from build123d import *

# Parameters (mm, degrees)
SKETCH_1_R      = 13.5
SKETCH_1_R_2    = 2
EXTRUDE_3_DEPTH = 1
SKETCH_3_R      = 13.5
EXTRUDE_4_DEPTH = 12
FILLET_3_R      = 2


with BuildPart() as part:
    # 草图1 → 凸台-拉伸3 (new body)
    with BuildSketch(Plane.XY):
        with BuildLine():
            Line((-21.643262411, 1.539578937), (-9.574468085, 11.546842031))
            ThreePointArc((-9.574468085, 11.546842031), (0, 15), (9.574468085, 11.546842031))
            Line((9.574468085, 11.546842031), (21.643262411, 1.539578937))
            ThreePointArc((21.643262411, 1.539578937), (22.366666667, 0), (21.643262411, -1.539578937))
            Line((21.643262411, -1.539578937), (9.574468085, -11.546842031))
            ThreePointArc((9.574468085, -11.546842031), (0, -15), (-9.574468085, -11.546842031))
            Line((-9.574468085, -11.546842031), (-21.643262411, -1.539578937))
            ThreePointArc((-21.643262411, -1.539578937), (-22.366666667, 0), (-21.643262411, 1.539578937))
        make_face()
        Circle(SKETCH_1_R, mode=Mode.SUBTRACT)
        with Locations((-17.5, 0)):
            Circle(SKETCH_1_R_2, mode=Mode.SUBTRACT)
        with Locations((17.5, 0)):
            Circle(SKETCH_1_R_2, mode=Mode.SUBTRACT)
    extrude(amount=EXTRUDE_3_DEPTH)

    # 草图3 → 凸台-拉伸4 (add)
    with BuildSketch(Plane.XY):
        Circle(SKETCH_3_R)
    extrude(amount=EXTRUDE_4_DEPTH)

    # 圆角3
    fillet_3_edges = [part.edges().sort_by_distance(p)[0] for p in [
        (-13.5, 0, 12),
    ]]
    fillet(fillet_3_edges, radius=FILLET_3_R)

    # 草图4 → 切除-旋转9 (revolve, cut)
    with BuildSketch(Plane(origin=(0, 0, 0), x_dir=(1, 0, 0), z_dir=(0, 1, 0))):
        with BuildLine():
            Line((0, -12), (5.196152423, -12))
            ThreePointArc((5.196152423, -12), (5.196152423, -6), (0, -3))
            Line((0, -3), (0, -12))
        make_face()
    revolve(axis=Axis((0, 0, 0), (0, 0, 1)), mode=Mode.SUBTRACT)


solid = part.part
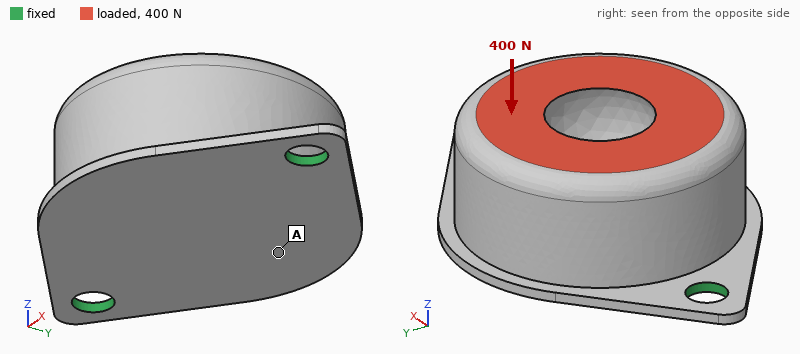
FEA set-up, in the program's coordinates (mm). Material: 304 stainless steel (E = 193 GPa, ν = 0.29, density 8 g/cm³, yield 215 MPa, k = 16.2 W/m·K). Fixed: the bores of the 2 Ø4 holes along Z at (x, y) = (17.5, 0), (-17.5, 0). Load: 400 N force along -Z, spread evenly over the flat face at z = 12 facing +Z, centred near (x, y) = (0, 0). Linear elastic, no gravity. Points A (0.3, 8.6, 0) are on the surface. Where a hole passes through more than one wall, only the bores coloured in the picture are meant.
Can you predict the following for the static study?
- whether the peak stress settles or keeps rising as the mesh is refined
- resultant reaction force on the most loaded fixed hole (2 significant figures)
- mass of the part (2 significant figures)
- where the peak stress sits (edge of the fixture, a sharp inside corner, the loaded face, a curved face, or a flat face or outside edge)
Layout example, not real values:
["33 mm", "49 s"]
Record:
["keeps rising", "240 N", "50 g", "edge of the fixture"]
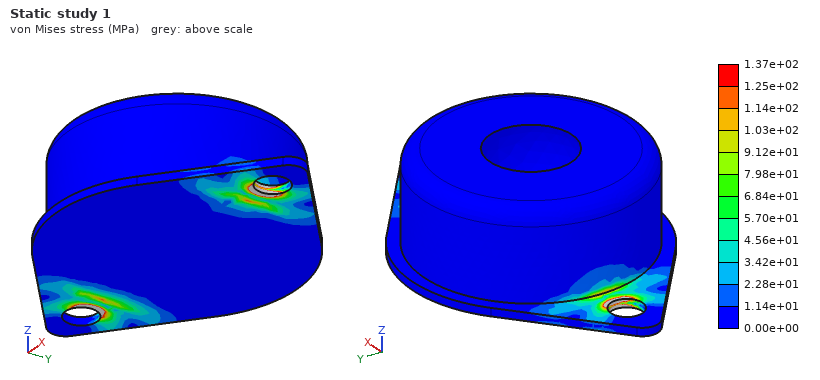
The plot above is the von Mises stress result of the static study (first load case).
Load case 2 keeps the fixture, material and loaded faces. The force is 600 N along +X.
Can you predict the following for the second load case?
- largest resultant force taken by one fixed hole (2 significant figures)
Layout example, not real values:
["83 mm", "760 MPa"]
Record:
["380 N"]
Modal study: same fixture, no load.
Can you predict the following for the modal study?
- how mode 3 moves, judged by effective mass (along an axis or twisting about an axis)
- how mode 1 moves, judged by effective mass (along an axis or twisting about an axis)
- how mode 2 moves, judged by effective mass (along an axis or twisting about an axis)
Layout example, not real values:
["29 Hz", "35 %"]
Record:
["along X", "along Y", "along Z"]
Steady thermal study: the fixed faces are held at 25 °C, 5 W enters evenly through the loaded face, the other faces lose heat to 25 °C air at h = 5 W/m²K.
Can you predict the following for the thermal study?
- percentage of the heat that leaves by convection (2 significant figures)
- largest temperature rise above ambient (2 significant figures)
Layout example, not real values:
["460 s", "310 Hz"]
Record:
["13 %", "65 K"]
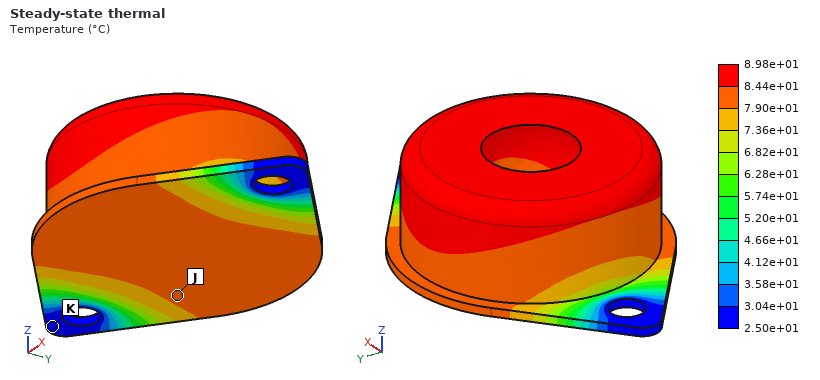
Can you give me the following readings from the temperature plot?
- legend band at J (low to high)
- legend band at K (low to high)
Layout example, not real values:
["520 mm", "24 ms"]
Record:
["7.90e+01 to 8.44e+01 °C", "2.50e+01 to 3.04e+01 °C"]
